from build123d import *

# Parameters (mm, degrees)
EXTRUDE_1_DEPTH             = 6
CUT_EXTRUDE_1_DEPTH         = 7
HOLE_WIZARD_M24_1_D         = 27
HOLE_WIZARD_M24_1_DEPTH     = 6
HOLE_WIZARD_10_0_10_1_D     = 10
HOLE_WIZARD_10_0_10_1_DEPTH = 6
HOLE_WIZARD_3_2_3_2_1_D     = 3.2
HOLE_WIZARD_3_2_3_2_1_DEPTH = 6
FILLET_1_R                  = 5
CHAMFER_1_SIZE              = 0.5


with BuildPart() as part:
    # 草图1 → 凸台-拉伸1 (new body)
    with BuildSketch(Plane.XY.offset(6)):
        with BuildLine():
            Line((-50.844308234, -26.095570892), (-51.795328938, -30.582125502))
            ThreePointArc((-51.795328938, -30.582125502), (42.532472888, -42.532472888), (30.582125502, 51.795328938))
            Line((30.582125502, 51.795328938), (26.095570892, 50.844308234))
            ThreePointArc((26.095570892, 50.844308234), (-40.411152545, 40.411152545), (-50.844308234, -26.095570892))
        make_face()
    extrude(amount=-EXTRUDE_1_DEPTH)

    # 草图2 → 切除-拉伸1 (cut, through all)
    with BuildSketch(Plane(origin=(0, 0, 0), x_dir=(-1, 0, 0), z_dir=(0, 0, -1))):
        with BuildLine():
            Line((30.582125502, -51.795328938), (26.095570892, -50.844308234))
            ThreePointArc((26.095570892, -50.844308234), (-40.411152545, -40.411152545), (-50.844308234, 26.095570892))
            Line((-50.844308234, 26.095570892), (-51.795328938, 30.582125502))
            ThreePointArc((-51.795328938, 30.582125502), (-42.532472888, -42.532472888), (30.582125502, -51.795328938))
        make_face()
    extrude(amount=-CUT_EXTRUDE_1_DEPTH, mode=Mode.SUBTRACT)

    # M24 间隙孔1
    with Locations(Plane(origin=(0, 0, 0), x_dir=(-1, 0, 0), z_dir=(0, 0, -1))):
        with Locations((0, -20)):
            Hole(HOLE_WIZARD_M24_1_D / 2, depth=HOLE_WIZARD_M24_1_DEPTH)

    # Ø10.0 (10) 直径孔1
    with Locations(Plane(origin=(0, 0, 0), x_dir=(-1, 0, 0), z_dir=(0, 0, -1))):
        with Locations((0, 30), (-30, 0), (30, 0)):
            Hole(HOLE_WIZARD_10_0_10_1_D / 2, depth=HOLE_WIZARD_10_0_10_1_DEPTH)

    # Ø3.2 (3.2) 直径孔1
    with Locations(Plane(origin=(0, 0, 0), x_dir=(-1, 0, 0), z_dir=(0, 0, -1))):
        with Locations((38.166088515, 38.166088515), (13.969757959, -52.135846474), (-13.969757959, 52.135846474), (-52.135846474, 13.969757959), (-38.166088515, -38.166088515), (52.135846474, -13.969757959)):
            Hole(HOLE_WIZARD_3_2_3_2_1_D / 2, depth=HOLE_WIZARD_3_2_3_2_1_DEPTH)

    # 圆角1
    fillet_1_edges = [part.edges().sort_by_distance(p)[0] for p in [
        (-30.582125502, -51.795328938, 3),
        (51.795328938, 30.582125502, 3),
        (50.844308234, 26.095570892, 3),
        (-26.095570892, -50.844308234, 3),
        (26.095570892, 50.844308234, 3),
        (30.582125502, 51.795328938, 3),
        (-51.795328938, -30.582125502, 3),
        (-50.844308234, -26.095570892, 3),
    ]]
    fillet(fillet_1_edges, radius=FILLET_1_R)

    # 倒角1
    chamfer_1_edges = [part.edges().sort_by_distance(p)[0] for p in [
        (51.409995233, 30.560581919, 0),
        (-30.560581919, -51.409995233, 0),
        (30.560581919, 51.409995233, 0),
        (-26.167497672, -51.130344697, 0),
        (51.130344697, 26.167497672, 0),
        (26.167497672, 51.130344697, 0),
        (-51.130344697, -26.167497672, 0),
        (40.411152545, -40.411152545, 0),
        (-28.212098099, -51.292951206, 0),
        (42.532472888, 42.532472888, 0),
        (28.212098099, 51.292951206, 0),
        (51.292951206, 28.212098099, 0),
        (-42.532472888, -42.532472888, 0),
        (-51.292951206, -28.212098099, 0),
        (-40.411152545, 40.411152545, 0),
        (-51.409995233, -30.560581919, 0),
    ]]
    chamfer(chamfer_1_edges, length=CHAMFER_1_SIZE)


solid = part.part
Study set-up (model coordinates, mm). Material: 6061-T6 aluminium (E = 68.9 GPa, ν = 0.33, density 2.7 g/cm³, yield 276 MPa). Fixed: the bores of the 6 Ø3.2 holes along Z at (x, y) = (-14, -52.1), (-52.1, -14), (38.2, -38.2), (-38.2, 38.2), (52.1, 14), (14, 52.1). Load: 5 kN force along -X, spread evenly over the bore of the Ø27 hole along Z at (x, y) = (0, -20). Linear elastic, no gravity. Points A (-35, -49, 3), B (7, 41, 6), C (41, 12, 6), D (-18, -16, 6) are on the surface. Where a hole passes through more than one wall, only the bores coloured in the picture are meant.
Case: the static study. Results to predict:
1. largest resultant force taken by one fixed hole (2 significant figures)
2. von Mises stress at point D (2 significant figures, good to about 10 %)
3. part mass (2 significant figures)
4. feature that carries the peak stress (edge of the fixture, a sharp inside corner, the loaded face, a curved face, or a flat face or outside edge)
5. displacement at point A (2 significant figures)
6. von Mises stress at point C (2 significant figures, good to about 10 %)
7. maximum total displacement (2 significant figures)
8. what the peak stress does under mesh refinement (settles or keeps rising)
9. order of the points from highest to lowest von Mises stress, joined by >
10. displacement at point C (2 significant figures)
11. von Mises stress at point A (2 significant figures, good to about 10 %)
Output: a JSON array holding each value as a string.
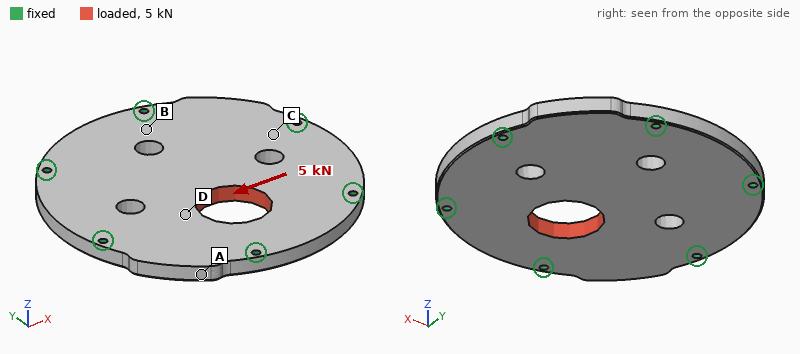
["1.3 kN", "11 MPa", "160 g", "edge of the fixture", "3.4 µm", "8.5 MPa", "7.1 µm", "keeps rising", "D > C > A > B", "1.7 µm", "4.8 MPa"]
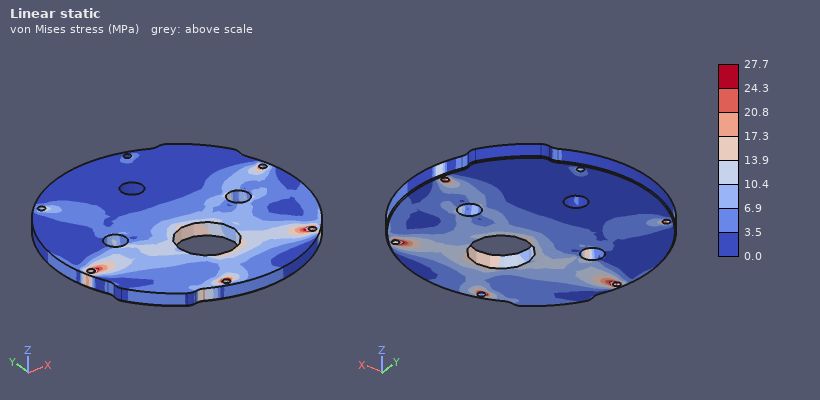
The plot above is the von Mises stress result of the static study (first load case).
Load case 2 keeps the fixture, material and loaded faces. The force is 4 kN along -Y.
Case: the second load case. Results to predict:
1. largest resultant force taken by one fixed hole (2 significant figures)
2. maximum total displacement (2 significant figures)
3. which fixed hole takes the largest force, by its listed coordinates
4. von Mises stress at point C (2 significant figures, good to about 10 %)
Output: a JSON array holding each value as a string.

["1.3 kN", "6.7 µm", "(-14, -52.1)", "3.1 MPa"]
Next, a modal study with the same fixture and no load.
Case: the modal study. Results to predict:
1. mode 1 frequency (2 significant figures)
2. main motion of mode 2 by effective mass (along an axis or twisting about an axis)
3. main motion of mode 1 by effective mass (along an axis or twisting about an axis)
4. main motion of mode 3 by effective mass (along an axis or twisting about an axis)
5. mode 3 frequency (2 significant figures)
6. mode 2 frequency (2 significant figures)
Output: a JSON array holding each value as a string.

["3600 Hz", "twisting about Y", "along Z", "twisting about X", "7600 Hz", "7100 Hz"]
